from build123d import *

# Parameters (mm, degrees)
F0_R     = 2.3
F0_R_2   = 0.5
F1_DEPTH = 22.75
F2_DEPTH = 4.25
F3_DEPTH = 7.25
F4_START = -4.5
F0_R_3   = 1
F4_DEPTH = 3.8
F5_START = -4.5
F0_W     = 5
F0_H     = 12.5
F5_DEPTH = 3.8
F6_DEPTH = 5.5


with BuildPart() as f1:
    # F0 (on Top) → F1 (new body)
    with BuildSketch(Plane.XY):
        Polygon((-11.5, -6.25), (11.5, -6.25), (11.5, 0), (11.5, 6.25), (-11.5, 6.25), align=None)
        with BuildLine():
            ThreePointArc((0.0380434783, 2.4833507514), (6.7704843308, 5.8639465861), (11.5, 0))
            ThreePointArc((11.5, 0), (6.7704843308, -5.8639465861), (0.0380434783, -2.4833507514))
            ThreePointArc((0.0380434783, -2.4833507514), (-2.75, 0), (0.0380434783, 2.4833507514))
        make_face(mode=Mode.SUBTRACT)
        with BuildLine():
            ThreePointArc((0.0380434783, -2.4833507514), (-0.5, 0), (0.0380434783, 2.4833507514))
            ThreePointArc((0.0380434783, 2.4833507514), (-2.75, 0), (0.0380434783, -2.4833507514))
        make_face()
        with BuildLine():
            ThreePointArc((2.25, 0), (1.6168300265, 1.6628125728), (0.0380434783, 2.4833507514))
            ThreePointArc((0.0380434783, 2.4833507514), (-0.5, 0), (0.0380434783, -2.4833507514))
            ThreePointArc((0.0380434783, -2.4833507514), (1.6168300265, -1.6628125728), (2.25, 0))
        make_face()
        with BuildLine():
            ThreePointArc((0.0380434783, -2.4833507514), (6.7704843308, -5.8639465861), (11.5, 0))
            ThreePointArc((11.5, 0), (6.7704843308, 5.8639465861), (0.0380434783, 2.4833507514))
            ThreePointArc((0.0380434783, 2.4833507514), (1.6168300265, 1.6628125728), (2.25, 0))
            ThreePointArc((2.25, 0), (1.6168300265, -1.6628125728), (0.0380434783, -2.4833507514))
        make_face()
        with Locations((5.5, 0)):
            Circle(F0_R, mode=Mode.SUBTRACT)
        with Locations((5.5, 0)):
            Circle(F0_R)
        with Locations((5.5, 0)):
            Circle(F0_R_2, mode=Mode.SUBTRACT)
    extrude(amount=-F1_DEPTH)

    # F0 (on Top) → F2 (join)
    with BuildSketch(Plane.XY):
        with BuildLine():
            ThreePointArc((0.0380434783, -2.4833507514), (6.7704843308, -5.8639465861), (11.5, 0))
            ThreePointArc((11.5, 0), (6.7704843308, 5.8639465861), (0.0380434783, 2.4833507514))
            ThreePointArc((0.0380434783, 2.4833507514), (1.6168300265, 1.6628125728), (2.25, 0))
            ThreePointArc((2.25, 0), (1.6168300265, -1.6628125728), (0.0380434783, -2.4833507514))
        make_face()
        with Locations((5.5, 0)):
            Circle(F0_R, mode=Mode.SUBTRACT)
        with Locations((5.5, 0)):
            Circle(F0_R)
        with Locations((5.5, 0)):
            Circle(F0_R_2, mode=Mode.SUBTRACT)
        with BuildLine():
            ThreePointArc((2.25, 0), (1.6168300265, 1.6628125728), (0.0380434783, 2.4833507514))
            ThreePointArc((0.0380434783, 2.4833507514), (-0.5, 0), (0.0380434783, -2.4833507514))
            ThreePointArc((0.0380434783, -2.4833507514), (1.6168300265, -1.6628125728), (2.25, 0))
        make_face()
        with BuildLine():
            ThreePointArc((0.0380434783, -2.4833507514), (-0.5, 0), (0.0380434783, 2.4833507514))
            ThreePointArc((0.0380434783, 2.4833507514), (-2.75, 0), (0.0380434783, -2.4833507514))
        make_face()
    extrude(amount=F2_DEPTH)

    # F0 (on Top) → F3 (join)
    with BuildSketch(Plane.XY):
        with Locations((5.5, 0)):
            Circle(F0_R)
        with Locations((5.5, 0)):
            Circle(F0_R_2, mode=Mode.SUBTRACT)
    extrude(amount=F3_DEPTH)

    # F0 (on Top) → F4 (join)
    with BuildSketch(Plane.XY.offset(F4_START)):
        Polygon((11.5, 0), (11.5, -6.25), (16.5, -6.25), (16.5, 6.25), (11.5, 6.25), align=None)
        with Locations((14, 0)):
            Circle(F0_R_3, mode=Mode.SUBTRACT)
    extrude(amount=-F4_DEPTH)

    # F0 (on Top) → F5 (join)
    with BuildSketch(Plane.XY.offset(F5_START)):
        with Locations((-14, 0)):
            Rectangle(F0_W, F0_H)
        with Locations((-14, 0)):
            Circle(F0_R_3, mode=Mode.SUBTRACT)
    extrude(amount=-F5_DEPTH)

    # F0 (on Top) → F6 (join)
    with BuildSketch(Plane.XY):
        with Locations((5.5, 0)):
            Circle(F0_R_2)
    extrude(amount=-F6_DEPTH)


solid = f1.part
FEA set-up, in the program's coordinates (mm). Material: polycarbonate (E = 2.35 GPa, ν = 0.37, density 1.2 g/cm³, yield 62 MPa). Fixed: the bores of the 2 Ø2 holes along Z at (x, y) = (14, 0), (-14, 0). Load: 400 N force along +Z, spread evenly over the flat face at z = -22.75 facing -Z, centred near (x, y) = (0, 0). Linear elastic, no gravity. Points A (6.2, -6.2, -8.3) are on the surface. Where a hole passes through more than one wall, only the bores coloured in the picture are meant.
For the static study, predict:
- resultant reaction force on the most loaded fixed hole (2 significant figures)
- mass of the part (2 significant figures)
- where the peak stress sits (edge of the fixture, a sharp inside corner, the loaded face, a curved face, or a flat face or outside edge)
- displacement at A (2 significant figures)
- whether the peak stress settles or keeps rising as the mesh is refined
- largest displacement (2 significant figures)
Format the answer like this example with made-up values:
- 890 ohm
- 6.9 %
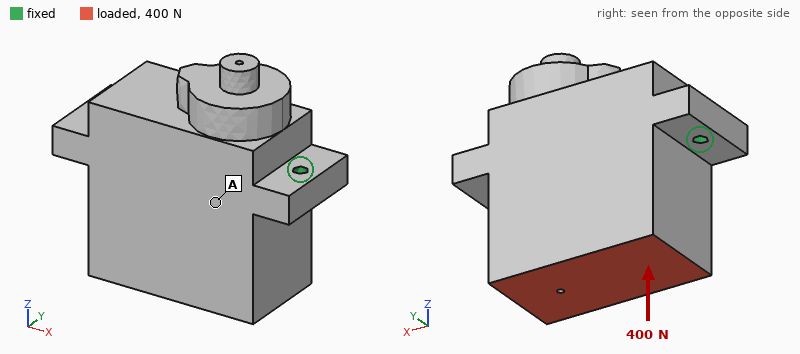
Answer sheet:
- 200 N
- 9.1 g
- edge of the fixture
- 44 µm
- keeps rising
- 50 µm
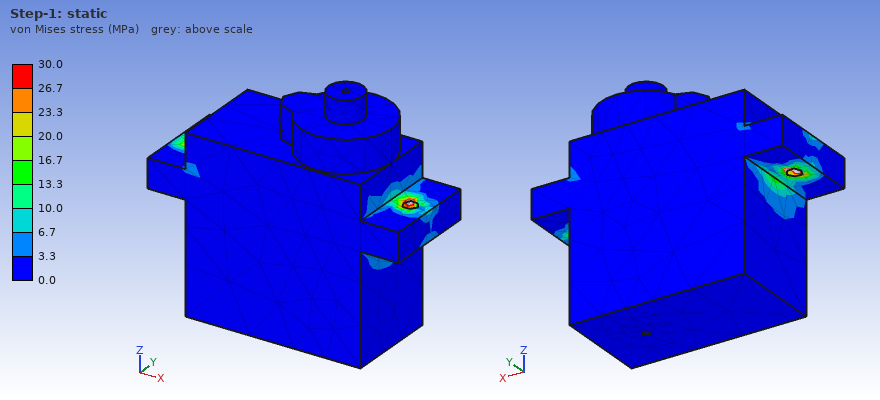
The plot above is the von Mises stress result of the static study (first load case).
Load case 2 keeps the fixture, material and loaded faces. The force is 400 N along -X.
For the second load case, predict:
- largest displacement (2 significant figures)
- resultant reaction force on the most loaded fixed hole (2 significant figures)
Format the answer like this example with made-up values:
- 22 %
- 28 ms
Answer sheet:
- 0.13 mm
- 320 N
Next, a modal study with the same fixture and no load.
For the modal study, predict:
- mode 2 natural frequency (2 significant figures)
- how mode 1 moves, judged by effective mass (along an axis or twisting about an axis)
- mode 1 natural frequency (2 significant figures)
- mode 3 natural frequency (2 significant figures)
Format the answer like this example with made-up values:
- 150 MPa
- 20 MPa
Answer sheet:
- 5200 Hz
- along Y
- 1700 Hz
- 5400 Hz
